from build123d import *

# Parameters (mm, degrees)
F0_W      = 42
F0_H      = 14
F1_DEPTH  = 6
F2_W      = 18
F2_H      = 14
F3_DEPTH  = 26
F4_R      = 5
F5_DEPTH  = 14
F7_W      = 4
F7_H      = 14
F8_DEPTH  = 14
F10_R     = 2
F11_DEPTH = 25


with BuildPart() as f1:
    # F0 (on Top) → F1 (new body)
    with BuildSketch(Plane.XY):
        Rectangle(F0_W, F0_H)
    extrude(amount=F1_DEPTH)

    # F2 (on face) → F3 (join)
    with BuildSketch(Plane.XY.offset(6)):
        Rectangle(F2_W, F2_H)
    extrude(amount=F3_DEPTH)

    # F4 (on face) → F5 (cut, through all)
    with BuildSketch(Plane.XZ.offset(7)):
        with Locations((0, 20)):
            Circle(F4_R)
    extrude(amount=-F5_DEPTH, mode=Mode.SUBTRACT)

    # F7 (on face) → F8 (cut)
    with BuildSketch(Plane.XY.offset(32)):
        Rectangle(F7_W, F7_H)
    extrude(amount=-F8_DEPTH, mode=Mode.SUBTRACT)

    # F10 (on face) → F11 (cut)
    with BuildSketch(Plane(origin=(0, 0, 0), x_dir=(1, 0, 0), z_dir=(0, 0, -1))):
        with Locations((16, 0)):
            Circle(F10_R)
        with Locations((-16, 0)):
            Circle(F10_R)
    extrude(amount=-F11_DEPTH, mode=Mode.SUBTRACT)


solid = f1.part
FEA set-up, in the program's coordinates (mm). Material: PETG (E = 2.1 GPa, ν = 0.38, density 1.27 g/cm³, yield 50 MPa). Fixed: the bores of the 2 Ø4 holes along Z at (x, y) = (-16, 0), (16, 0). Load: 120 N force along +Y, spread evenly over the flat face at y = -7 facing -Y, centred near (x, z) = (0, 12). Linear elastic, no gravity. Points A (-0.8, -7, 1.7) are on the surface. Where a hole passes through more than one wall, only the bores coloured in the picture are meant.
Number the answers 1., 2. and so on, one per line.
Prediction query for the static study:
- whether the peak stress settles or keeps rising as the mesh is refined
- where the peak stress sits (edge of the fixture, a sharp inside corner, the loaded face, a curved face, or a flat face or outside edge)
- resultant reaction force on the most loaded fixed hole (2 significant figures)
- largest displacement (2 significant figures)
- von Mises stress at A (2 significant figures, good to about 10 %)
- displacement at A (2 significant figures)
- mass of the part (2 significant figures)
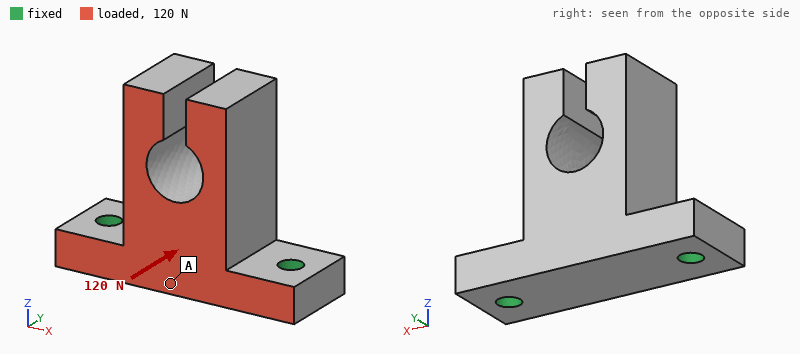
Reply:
1. keeps rising
2. edge of the fixture
3. 60 N
4. 0.25 mm
5. 1.6 MPa
6. 0.049 mm
7. 11 g
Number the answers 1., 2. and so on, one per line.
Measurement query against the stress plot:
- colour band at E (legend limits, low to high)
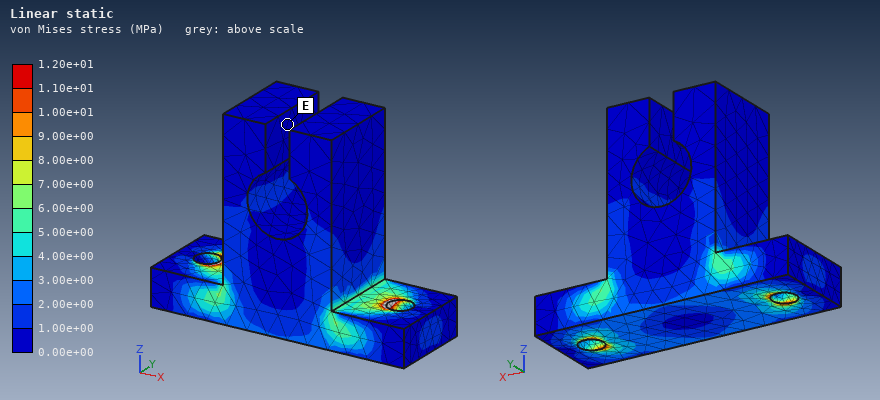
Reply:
1. 0.00e+00 to 1.00e+00 MPa
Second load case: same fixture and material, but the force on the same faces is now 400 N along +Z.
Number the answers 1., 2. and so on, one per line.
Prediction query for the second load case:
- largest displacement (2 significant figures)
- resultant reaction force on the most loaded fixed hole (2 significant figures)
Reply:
1. 0.53 mm
2. 210 N
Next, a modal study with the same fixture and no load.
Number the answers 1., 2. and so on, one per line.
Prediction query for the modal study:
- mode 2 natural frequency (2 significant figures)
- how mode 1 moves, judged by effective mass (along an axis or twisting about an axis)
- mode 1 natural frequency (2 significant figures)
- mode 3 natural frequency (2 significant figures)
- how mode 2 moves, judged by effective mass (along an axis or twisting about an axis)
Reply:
1. 1900 Hz
2. along Y
3. 1300 Hz
4. 2200 Hz
5. along X
